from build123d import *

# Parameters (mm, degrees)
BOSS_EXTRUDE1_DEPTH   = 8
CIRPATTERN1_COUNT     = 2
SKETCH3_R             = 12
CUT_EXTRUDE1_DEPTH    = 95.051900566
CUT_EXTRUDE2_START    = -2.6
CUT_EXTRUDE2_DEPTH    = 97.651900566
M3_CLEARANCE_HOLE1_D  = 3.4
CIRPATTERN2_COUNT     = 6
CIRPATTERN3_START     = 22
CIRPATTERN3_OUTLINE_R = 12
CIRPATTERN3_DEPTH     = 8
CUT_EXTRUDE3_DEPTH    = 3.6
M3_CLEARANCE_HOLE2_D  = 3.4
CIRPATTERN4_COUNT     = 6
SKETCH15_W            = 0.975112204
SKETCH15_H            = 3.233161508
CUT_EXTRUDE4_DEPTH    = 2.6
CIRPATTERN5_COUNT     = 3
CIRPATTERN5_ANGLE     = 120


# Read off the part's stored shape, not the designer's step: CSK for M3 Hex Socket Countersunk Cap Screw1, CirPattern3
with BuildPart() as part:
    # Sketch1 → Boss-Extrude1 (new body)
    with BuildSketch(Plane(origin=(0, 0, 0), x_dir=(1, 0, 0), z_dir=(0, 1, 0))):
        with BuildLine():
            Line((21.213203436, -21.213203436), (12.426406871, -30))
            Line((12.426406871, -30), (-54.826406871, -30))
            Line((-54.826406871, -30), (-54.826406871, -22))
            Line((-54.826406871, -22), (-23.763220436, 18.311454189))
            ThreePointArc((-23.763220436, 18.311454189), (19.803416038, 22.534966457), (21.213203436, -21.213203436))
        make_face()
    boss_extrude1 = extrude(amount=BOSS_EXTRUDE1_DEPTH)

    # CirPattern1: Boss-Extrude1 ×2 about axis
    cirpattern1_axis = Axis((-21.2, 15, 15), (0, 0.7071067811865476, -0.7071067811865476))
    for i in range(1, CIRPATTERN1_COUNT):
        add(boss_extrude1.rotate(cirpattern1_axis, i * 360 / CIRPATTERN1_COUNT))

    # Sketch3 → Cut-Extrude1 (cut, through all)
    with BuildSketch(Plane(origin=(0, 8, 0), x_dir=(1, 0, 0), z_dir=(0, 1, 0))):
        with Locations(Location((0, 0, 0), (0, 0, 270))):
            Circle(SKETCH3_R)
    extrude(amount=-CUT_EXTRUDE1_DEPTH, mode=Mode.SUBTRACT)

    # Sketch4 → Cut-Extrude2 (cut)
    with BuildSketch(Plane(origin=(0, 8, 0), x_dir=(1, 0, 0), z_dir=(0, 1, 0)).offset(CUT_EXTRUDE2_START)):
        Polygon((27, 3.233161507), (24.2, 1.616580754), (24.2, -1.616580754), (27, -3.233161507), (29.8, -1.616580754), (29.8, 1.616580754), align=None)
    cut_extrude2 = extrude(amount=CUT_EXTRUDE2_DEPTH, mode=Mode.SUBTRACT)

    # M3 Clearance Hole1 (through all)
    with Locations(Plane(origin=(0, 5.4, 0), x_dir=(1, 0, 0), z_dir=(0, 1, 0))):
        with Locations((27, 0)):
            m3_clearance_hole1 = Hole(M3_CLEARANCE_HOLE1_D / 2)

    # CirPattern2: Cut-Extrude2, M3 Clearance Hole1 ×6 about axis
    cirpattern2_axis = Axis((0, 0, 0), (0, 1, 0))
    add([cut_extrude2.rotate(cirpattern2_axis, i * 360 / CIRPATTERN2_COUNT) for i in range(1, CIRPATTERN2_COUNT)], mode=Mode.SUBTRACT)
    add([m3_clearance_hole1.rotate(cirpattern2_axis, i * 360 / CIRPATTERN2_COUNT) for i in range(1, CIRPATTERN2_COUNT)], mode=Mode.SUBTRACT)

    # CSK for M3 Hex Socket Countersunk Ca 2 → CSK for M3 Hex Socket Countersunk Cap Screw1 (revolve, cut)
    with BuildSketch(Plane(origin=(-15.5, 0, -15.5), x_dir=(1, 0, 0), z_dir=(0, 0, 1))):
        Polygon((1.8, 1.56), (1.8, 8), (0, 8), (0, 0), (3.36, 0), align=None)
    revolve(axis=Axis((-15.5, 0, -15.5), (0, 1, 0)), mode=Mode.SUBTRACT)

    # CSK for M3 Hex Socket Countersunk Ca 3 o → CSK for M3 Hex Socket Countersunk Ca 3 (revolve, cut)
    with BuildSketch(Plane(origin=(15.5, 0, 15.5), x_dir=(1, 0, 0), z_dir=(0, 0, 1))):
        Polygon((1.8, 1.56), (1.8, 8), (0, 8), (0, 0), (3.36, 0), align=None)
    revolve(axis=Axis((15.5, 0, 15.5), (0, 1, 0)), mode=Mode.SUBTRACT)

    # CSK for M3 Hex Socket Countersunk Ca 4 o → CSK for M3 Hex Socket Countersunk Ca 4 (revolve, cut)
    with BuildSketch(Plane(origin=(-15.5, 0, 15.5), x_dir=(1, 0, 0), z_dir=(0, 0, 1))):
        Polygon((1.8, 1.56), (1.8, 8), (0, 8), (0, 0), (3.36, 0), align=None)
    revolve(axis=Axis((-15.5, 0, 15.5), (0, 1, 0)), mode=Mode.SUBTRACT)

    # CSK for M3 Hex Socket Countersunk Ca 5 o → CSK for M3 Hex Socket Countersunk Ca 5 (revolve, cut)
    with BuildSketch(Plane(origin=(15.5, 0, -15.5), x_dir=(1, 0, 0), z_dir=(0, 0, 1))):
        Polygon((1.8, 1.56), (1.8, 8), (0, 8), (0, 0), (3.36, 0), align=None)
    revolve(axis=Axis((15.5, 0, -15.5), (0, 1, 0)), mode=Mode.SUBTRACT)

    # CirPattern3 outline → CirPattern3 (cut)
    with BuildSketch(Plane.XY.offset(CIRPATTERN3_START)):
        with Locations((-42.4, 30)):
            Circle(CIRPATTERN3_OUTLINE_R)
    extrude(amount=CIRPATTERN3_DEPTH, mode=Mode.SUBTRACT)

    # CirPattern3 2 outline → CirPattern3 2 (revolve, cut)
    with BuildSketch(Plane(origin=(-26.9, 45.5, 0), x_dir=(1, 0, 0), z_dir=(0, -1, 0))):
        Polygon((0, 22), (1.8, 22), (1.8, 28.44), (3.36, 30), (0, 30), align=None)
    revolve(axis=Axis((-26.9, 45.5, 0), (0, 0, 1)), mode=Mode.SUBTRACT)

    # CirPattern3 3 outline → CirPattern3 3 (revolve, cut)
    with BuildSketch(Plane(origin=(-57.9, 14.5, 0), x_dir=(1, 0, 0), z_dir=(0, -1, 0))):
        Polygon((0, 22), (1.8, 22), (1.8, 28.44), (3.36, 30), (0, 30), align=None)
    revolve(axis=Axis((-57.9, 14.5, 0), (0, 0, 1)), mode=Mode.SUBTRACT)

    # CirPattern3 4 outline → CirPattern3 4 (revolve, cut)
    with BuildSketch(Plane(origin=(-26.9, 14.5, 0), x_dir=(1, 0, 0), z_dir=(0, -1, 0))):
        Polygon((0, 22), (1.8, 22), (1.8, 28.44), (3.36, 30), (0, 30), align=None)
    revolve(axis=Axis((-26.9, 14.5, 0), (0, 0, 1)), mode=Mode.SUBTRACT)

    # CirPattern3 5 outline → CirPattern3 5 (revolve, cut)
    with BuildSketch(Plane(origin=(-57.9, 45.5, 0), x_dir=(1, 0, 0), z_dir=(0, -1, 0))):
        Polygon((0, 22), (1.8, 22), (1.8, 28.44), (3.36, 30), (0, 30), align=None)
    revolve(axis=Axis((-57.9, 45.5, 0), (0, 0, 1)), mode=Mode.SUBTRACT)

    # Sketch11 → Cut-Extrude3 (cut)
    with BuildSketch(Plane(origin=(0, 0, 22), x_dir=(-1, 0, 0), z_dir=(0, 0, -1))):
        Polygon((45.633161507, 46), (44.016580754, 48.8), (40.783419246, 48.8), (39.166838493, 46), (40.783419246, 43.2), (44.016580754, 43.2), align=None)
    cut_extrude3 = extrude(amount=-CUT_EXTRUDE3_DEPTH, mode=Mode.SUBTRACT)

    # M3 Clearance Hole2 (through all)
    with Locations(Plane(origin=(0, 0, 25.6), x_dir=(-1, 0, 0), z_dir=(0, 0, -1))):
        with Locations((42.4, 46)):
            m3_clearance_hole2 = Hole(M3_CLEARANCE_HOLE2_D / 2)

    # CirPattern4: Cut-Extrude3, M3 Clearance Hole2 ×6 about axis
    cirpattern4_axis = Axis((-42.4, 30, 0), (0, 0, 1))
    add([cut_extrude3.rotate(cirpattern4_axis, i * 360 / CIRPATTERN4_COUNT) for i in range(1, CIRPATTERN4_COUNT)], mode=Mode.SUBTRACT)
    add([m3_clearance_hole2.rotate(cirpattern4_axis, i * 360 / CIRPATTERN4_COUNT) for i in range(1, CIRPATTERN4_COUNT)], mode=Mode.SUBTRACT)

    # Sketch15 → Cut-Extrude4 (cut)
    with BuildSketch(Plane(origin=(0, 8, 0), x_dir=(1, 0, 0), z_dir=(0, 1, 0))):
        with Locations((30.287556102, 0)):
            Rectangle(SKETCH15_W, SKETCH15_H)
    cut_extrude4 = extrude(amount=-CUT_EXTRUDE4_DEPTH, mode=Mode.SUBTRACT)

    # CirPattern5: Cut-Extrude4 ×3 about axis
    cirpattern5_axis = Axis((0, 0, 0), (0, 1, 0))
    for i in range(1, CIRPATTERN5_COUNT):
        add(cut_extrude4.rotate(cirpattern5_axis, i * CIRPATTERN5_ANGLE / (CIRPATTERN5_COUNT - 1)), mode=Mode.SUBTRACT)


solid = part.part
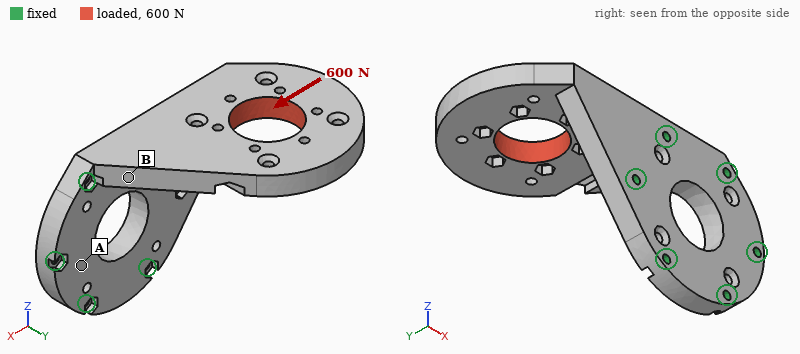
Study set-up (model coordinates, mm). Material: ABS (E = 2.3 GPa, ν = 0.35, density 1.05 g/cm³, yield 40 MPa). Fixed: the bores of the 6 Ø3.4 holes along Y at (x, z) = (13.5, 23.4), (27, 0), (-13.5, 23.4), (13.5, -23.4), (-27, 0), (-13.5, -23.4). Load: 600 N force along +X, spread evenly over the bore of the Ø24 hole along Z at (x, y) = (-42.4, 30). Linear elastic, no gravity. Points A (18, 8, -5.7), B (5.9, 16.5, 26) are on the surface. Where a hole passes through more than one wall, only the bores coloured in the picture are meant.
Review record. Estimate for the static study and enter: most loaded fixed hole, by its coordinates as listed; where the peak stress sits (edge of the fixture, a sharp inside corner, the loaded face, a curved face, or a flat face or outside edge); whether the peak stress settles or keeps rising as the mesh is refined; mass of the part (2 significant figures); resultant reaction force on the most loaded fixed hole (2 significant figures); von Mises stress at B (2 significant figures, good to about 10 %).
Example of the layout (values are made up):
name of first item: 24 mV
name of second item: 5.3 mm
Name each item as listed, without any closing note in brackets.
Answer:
most loaded fixed hole, by its coordinates as listed: (13.5, 23.4)
where the peak stress sits: edge of the fixture
whether the peak stress settles or keeps rising as the mesh is refined: keeps rising
mass of the part: 46 g
resultant reaction force on the most loaded fixed hole: 620 N
von Mises stress at B: 11 MPa
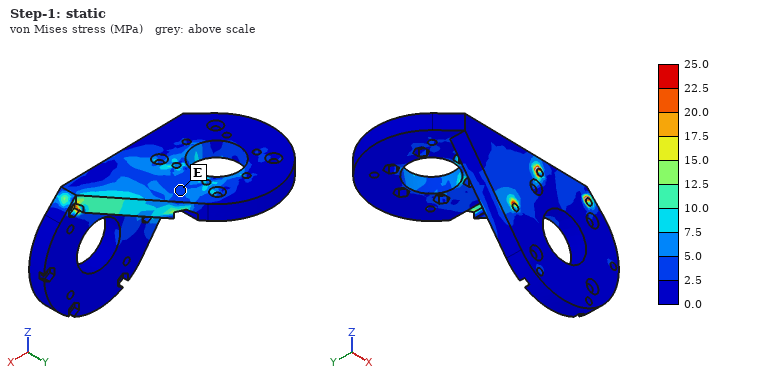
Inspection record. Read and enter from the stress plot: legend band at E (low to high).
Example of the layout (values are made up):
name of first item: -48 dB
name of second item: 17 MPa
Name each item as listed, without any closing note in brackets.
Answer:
legend band at E: 2.5 to 5.0 MPa
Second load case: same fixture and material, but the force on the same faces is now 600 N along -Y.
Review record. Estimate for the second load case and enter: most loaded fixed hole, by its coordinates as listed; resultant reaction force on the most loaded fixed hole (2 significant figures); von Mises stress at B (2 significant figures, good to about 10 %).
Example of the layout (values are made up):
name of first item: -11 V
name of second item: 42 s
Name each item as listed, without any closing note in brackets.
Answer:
most loaded fixed hole, by its coordinates as listed: (-13.5, 23.4)
resultant reaction force on the most loaded fixed hole: 1.0 kN
von Mises stress at B: 12 MPa
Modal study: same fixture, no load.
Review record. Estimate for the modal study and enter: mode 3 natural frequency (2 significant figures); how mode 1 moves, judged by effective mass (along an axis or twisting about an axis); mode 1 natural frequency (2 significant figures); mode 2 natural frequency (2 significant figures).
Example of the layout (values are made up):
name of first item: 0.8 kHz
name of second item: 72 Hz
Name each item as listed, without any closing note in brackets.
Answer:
mode 3 natural frequency: 1300 Hz
how mode 1 moves, judged by effective mass: along Z
mode 1 natural frequency: 480 Hz
mode 2 natural frequency: 870 Hz
